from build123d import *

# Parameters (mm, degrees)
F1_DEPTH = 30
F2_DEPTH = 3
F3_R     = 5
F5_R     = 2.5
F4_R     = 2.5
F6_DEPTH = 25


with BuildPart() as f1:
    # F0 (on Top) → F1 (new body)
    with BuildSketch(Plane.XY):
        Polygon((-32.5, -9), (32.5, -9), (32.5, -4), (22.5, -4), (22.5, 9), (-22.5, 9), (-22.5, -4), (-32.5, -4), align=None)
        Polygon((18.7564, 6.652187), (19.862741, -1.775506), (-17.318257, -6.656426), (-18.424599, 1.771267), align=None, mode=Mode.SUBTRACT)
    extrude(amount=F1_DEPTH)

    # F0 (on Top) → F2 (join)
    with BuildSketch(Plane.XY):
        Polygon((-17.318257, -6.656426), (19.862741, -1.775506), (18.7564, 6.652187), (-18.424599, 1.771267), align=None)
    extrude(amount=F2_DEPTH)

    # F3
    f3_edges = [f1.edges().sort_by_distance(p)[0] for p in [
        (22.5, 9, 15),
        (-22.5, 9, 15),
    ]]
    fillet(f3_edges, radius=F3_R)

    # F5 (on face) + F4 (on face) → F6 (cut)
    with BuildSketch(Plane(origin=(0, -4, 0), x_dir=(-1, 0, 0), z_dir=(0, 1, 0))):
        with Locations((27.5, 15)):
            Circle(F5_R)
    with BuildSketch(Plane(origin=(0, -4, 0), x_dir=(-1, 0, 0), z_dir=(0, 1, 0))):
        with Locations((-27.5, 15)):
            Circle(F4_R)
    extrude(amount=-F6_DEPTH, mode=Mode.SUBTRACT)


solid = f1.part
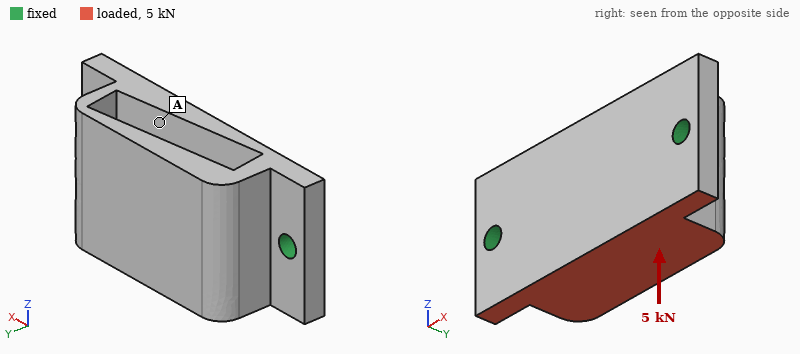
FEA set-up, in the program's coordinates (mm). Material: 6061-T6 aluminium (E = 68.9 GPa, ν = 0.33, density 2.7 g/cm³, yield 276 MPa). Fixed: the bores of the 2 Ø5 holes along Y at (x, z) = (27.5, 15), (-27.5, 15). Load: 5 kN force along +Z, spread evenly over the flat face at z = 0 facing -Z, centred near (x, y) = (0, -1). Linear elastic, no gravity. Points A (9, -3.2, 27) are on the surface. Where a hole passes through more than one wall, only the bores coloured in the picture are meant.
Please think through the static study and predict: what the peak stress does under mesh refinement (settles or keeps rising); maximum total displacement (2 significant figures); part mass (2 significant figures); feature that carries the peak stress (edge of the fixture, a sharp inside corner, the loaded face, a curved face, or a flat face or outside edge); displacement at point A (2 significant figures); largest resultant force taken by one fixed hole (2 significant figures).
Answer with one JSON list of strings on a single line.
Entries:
["keeps rising", "86 µm", "49 g", "edge of the fixture", "52 µm", "2.5 kN"]
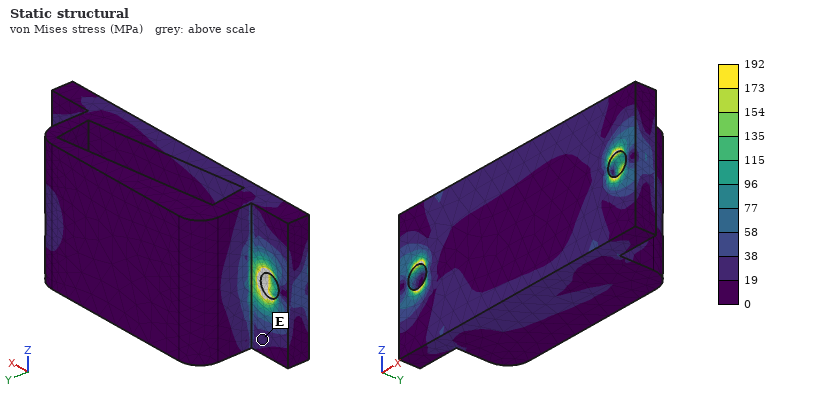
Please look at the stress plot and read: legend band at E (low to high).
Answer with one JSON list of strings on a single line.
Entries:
["19 to 38 MPa"]
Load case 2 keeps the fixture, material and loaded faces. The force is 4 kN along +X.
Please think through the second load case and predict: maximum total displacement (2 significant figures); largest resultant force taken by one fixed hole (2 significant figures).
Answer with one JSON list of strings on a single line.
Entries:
["16 µm", "2.3 kN"]
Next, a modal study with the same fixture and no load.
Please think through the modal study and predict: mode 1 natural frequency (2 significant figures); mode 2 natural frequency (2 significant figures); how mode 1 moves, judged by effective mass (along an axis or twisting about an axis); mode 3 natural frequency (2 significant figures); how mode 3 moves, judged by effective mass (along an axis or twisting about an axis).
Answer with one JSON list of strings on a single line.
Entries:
["5400 Hz", "8400 Hz", "along Z", "9800 Hz", "along Y"]
